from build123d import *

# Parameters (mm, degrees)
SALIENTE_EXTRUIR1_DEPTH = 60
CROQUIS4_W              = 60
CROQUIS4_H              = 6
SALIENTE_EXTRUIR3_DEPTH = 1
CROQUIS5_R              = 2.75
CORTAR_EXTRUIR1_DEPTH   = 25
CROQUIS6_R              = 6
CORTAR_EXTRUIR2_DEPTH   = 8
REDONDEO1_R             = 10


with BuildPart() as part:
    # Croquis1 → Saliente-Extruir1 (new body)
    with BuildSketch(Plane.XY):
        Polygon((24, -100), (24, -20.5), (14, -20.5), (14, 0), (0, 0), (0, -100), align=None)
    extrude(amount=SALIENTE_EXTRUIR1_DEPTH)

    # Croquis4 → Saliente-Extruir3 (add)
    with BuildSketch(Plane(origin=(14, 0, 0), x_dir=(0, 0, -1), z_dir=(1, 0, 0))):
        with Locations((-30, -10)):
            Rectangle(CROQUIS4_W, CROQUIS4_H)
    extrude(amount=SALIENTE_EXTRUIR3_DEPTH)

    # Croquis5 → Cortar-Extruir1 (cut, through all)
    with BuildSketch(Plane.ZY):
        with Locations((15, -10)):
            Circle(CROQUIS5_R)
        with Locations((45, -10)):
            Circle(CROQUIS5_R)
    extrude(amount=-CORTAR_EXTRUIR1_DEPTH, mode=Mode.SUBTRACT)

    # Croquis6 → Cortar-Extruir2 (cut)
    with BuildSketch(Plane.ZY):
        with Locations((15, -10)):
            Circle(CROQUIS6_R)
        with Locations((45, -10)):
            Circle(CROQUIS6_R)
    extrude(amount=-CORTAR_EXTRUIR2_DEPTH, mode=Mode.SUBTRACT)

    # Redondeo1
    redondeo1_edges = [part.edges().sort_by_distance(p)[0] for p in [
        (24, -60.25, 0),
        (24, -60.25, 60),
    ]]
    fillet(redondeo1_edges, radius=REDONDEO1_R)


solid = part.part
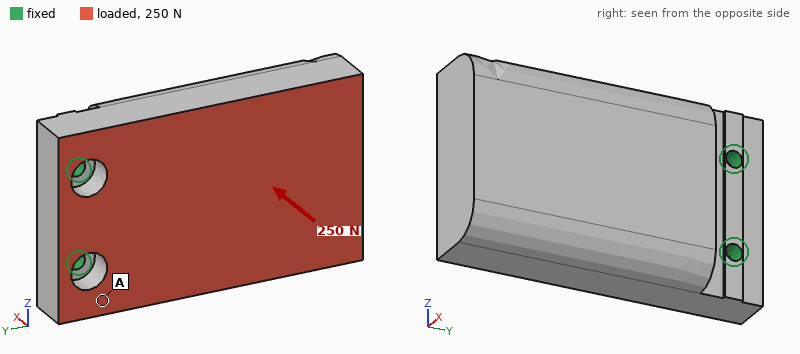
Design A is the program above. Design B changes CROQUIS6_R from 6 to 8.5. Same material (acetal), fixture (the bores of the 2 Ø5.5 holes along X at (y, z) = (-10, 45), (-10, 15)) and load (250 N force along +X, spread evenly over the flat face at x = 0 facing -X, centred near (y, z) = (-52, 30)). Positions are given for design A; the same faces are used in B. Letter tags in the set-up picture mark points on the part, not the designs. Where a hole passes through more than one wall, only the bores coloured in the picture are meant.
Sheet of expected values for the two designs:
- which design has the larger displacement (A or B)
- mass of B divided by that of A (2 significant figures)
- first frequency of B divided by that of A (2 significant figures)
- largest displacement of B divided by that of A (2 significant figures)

B
0.99
0.94
1.2
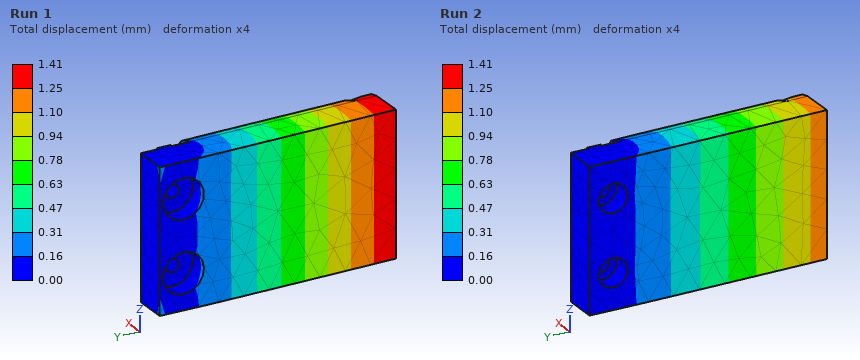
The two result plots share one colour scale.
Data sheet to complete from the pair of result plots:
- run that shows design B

Run 1
